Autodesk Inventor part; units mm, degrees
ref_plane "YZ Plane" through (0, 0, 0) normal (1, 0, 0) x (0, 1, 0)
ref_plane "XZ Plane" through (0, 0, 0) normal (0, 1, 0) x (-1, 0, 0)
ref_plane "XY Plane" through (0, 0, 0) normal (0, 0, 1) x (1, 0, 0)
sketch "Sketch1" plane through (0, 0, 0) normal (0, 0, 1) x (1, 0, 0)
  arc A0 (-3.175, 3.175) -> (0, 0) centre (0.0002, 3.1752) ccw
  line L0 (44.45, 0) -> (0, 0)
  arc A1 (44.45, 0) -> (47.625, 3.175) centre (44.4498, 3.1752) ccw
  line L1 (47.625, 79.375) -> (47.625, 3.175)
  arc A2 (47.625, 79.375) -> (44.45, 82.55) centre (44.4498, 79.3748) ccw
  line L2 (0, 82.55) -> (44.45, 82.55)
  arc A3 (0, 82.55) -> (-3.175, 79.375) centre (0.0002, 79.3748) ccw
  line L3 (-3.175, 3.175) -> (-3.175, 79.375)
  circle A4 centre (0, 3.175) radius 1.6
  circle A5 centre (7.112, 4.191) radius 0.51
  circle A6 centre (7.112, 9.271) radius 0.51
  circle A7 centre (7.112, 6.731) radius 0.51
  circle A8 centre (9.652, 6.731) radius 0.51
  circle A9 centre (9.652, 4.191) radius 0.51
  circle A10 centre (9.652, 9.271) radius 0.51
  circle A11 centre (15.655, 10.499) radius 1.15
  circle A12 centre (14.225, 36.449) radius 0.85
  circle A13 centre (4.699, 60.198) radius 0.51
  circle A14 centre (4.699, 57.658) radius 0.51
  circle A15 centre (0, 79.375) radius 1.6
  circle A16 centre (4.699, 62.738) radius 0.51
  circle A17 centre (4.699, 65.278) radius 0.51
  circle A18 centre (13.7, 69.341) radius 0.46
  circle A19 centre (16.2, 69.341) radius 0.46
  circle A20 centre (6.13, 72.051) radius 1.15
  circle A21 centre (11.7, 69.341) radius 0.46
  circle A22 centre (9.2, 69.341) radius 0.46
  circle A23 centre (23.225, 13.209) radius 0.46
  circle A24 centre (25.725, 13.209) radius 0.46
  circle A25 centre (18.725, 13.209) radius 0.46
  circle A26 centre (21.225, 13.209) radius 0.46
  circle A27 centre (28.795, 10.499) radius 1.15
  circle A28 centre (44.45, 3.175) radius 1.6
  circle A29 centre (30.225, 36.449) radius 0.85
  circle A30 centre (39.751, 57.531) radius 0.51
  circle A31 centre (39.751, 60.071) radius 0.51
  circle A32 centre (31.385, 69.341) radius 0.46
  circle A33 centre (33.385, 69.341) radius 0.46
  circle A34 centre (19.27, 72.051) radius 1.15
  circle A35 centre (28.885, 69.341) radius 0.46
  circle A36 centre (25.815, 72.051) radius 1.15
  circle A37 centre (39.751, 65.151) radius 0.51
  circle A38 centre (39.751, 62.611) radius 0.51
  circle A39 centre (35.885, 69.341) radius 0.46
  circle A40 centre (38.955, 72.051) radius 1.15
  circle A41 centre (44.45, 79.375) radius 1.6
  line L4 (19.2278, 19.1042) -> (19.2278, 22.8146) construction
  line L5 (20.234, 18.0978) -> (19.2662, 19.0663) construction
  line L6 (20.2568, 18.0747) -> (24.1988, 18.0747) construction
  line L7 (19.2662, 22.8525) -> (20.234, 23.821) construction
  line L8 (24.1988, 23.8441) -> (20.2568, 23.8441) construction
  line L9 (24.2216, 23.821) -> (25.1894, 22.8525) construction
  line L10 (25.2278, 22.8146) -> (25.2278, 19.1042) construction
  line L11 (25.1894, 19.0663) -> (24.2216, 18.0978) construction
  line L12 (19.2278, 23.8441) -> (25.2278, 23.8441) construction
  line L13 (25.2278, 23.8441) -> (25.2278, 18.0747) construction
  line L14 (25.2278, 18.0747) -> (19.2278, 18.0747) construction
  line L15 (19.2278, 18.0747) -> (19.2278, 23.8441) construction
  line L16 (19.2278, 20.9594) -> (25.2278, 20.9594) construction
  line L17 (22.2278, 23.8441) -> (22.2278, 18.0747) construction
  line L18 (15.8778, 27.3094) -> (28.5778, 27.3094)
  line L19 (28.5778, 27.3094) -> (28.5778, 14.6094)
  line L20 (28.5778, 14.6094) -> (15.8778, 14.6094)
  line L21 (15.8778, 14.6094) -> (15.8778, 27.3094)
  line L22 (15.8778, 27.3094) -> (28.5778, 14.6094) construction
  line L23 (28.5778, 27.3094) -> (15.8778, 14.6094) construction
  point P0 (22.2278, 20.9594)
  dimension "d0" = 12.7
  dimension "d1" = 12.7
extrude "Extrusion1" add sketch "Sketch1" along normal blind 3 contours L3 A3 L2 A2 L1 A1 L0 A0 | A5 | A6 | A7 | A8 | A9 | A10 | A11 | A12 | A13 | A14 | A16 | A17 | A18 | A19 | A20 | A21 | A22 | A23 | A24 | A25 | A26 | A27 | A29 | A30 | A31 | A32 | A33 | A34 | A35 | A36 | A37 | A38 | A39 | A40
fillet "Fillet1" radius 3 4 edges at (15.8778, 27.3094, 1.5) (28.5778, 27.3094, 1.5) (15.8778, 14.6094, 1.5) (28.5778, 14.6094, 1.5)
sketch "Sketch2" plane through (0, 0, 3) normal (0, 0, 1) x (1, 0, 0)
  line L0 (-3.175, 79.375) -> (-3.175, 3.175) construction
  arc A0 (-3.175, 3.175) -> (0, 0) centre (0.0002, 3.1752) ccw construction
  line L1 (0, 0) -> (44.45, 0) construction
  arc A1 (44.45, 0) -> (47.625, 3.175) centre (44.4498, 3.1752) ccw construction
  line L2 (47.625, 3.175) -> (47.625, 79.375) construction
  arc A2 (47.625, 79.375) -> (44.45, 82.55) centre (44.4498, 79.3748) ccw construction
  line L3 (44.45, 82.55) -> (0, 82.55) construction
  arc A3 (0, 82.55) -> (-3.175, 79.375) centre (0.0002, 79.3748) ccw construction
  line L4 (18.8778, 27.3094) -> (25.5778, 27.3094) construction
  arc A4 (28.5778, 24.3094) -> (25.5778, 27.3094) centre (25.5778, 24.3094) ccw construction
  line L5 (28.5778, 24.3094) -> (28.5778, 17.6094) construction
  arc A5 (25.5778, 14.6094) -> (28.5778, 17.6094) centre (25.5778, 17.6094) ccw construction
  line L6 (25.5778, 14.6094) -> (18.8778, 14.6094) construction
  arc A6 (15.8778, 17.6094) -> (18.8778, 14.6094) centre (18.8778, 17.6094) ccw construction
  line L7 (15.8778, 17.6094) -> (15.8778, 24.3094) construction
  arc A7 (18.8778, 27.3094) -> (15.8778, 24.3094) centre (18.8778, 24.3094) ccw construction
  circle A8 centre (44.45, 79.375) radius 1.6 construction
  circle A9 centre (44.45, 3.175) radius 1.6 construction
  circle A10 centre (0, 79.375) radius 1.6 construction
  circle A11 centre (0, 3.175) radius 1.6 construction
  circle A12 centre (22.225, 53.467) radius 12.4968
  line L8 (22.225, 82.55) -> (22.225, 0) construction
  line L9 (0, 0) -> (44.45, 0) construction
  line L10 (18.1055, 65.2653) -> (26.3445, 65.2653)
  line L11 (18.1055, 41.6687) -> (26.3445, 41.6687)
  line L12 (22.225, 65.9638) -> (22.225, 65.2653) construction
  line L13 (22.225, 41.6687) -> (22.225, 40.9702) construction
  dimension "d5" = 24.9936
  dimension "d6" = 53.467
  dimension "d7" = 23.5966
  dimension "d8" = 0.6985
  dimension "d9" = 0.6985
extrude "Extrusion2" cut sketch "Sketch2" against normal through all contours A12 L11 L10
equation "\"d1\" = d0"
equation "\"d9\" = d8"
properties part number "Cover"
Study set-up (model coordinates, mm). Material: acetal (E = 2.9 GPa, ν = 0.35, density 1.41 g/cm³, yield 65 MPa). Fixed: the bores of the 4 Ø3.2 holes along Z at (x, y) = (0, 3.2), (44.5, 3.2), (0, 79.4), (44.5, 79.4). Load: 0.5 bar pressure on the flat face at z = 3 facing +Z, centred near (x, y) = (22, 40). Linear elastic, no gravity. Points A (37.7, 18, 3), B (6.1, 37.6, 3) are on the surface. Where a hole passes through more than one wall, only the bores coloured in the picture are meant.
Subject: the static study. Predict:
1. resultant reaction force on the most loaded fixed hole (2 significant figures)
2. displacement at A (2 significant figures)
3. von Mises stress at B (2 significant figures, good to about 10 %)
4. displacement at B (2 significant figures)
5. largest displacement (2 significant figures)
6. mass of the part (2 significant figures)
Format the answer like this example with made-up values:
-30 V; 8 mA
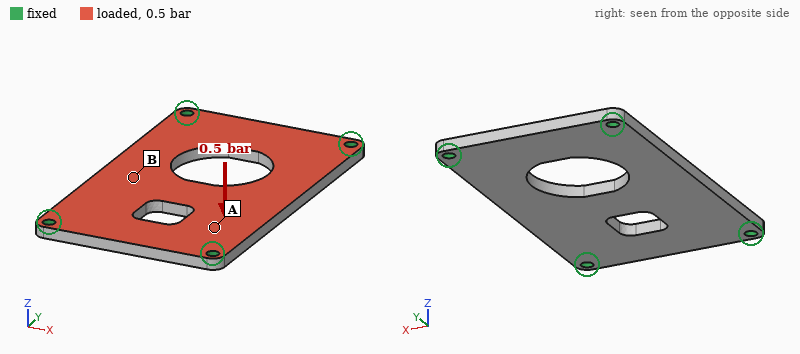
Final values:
45 N; 0.43 mm; 8.0 MPa; 0.90 mm; 1.1 mm; 15 g
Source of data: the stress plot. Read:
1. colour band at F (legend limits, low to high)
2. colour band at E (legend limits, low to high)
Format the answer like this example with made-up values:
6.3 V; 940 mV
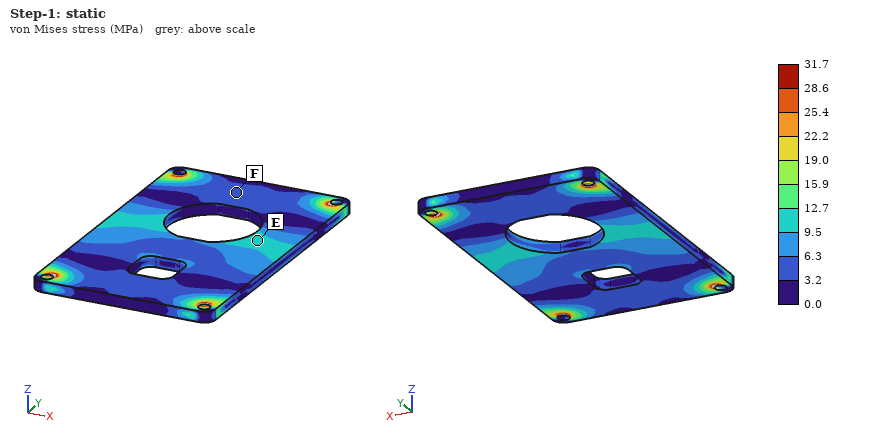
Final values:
3.2 to 6.3 MPa; 9.5 to 12.7 MPa
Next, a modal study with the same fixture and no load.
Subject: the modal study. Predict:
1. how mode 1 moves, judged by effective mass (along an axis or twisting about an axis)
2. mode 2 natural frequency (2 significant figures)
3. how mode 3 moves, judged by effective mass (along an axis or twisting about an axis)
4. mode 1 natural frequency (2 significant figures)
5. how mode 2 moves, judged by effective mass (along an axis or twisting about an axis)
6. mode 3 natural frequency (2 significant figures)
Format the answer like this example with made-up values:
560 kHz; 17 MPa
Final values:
along Z; 990 Hz; twisting about X; 650 Hz; twisting about Y; 1600 Hz
